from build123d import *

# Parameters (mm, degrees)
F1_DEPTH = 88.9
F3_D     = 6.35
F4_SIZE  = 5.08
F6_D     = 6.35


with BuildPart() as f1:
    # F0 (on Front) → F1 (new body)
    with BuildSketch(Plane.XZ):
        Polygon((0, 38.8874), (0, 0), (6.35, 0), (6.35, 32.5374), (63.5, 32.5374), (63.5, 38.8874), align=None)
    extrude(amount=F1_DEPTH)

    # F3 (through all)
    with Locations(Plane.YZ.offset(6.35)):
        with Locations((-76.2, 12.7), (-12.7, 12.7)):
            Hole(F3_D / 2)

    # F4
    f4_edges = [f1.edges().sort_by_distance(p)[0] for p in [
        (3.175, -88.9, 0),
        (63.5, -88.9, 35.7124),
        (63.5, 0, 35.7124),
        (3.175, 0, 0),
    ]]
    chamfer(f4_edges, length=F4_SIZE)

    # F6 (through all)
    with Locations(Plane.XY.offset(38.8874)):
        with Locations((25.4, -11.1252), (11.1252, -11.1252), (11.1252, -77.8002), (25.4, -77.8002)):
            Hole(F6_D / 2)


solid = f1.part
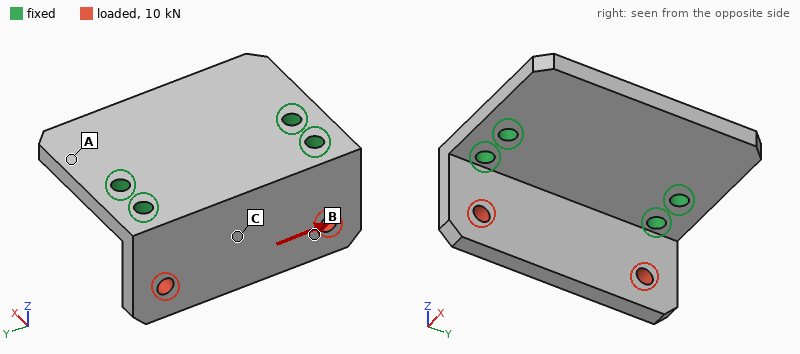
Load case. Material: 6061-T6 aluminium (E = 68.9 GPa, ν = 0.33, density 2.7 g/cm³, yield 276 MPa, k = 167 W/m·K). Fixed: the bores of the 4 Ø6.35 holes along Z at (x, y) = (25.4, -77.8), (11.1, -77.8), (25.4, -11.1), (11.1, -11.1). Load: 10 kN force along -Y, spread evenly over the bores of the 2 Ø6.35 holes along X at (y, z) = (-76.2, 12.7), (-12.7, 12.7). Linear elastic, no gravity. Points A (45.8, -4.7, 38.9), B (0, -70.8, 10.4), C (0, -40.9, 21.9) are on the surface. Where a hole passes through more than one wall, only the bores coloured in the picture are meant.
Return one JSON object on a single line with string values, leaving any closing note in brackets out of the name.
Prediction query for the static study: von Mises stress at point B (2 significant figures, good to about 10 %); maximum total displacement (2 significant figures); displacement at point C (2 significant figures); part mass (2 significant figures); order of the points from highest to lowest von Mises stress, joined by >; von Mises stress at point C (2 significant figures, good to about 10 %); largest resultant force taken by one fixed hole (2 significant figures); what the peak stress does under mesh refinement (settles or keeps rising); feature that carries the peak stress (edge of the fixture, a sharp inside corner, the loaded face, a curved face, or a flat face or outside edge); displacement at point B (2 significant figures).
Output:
{"von Mises stress at point B": "46 MPa", "maximum total displacement": "71 µm", "displacement at point C": "21 µm", "part mass": "140 g", "order of the points from highest to lowest von Mises stress, joined by >": "B > C > A", "von Mises stress at point C": "22 MPa", "largest resultant force taken by one fixed hole": "5.4 kN", "what the peak stress does under mesh refinement": "keeps rising", "feature that carries the peak stress": "edge of the fixture", "displacement at point B": "47 µm"}
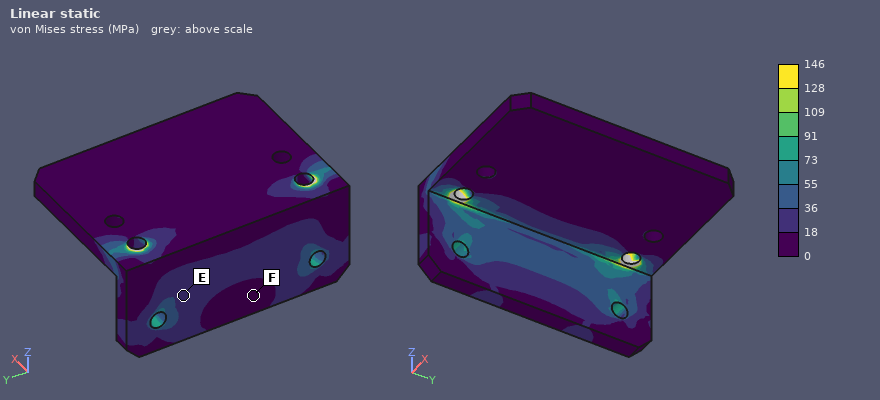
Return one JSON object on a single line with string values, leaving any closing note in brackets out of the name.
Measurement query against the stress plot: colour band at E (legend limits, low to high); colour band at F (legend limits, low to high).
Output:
{"colour band at E": "18 to 36 MPa", "colour band at F": "0 to 18 MPa"}
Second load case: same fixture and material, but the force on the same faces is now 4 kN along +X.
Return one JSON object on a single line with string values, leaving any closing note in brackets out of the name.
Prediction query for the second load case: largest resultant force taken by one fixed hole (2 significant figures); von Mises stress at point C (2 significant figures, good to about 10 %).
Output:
{"largest resultant force taken by one fixed hole": "1.9 kN", "von Mises stress at point C": "50 MPa"}
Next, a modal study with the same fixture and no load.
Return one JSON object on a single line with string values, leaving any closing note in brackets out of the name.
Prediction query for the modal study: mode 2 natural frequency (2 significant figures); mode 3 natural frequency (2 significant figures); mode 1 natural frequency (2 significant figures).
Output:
{"mode 2 natural frequency": "3200 Hz", "mode 3 natural frequency": "4900 Hz", "mode 1 natural frequency": "2900 Hz"}
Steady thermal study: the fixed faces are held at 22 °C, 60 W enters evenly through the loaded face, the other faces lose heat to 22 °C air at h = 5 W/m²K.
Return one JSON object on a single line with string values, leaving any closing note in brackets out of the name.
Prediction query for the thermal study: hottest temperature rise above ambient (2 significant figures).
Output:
{"hottest temperature rise above ambient": "29 K"}
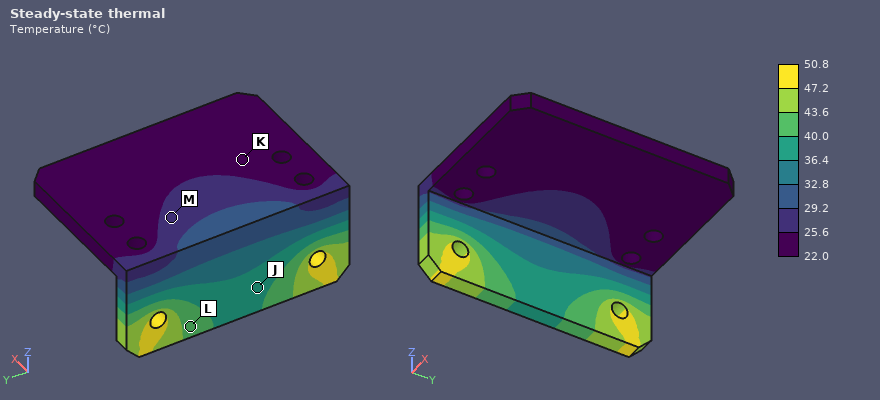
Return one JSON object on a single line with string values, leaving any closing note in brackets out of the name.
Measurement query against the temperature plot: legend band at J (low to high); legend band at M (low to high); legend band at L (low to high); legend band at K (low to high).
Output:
{"legend band at J": "36.4 to 40.0 °C", "legend band at M": "25.6 to 29.2 °C", "legend band at L": "40.0 to 43.6 °C", "legend band at K": "22.0 to 25.6 °C"}
